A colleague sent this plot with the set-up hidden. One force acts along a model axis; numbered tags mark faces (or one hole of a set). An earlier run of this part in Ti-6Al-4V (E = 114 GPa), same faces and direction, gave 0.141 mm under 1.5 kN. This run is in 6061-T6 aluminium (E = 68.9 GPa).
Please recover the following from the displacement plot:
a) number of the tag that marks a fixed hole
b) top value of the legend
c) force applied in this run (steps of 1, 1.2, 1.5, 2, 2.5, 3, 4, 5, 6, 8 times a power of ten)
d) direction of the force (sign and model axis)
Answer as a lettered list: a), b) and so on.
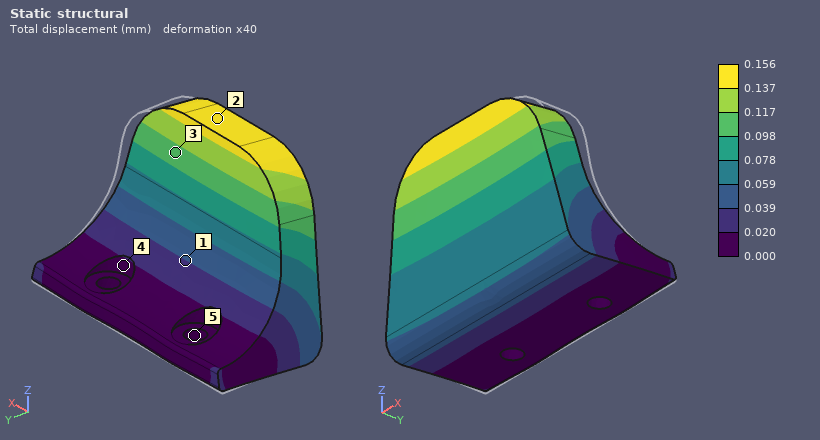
a) 5
b) 0.156 mm
c) 1 kN
d) -Y
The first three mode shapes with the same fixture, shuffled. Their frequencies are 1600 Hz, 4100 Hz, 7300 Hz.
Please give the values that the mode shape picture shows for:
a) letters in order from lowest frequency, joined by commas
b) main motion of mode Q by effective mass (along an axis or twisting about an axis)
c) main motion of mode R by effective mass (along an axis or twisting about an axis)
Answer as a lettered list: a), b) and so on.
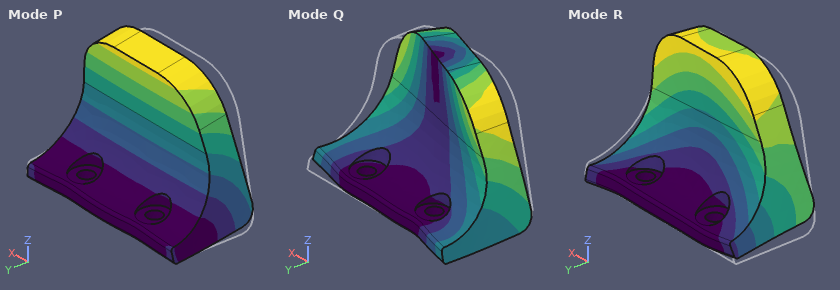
a) P, R, Q
b) along X
c) along X
